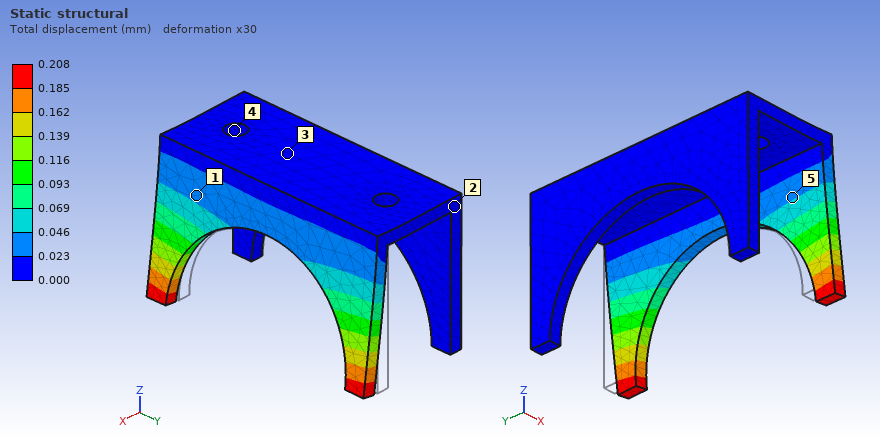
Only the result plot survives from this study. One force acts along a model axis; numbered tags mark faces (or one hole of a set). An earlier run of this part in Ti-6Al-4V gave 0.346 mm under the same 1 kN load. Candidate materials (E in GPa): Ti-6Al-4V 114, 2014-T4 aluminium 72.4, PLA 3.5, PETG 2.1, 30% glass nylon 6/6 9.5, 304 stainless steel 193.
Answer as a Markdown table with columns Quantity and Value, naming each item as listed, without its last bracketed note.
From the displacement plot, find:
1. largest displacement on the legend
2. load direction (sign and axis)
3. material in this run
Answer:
| Quantity | Value |
|---|---|
| largest displacement on the legend | 0.208 mm |
| load direction | +X |
| material in this run | 304 stainless steel |
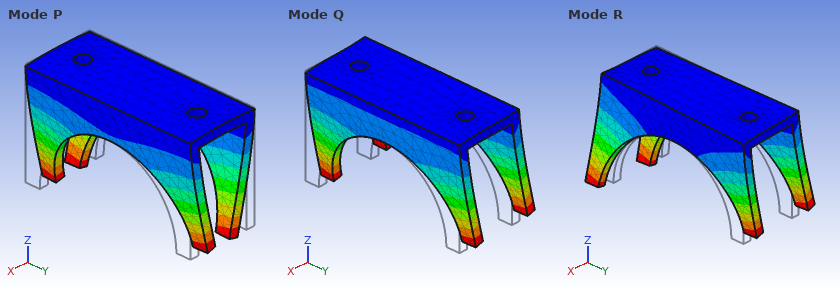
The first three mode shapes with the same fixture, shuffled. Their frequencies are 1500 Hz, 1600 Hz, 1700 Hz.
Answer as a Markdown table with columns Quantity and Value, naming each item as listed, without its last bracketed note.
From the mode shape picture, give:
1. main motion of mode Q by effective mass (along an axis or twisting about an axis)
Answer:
| Quantity | Value |
|---|---|
| main motion of mode Q by effective mass | along X |
